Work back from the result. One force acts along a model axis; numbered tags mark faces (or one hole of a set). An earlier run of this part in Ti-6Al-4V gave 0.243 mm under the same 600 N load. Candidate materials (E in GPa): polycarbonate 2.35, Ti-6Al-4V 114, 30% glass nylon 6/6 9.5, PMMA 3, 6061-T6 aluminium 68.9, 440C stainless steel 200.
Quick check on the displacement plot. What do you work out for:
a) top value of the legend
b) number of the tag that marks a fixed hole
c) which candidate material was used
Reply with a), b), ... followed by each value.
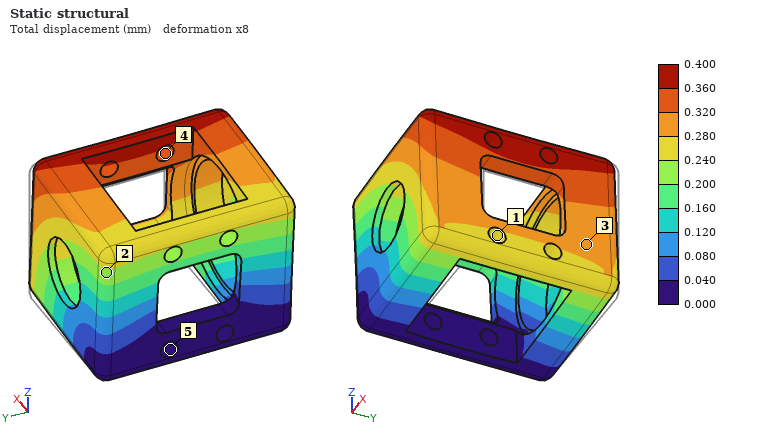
a) 0.400 mm
b) 5
c) 6061-T6 aluminium
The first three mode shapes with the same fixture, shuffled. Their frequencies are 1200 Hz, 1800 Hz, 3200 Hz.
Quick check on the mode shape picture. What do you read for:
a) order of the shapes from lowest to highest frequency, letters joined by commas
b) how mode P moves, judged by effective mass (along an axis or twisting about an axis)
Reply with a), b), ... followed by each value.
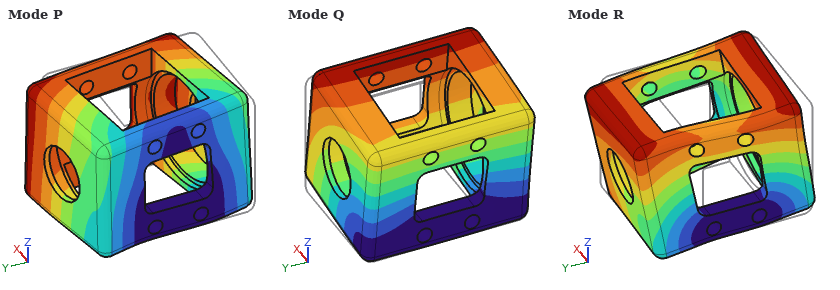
a) Q, P, R
b) along Y
